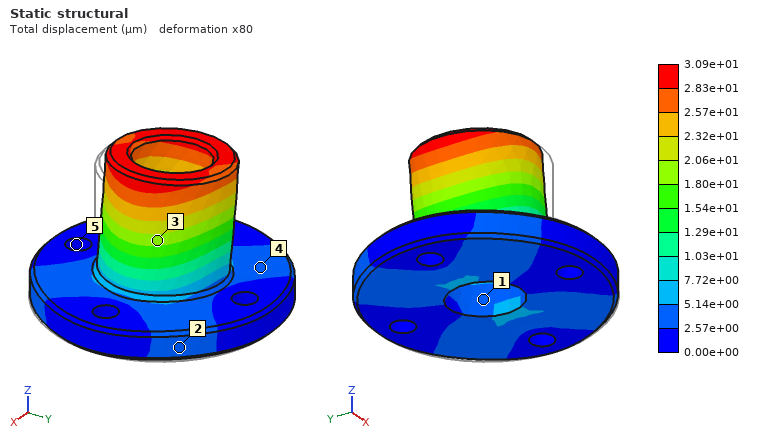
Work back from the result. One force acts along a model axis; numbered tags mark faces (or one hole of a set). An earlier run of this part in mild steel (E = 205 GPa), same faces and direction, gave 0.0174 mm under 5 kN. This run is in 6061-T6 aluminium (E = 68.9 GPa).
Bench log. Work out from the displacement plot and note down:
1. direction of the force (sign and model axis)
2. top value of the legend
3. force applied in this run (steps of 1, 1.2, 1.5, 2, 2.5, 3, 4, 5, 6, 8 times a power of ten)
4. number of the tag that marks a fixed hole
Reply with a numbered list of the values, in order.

1. -X
2. 3.09e+01 µm
3. 3 kN
4. 5
